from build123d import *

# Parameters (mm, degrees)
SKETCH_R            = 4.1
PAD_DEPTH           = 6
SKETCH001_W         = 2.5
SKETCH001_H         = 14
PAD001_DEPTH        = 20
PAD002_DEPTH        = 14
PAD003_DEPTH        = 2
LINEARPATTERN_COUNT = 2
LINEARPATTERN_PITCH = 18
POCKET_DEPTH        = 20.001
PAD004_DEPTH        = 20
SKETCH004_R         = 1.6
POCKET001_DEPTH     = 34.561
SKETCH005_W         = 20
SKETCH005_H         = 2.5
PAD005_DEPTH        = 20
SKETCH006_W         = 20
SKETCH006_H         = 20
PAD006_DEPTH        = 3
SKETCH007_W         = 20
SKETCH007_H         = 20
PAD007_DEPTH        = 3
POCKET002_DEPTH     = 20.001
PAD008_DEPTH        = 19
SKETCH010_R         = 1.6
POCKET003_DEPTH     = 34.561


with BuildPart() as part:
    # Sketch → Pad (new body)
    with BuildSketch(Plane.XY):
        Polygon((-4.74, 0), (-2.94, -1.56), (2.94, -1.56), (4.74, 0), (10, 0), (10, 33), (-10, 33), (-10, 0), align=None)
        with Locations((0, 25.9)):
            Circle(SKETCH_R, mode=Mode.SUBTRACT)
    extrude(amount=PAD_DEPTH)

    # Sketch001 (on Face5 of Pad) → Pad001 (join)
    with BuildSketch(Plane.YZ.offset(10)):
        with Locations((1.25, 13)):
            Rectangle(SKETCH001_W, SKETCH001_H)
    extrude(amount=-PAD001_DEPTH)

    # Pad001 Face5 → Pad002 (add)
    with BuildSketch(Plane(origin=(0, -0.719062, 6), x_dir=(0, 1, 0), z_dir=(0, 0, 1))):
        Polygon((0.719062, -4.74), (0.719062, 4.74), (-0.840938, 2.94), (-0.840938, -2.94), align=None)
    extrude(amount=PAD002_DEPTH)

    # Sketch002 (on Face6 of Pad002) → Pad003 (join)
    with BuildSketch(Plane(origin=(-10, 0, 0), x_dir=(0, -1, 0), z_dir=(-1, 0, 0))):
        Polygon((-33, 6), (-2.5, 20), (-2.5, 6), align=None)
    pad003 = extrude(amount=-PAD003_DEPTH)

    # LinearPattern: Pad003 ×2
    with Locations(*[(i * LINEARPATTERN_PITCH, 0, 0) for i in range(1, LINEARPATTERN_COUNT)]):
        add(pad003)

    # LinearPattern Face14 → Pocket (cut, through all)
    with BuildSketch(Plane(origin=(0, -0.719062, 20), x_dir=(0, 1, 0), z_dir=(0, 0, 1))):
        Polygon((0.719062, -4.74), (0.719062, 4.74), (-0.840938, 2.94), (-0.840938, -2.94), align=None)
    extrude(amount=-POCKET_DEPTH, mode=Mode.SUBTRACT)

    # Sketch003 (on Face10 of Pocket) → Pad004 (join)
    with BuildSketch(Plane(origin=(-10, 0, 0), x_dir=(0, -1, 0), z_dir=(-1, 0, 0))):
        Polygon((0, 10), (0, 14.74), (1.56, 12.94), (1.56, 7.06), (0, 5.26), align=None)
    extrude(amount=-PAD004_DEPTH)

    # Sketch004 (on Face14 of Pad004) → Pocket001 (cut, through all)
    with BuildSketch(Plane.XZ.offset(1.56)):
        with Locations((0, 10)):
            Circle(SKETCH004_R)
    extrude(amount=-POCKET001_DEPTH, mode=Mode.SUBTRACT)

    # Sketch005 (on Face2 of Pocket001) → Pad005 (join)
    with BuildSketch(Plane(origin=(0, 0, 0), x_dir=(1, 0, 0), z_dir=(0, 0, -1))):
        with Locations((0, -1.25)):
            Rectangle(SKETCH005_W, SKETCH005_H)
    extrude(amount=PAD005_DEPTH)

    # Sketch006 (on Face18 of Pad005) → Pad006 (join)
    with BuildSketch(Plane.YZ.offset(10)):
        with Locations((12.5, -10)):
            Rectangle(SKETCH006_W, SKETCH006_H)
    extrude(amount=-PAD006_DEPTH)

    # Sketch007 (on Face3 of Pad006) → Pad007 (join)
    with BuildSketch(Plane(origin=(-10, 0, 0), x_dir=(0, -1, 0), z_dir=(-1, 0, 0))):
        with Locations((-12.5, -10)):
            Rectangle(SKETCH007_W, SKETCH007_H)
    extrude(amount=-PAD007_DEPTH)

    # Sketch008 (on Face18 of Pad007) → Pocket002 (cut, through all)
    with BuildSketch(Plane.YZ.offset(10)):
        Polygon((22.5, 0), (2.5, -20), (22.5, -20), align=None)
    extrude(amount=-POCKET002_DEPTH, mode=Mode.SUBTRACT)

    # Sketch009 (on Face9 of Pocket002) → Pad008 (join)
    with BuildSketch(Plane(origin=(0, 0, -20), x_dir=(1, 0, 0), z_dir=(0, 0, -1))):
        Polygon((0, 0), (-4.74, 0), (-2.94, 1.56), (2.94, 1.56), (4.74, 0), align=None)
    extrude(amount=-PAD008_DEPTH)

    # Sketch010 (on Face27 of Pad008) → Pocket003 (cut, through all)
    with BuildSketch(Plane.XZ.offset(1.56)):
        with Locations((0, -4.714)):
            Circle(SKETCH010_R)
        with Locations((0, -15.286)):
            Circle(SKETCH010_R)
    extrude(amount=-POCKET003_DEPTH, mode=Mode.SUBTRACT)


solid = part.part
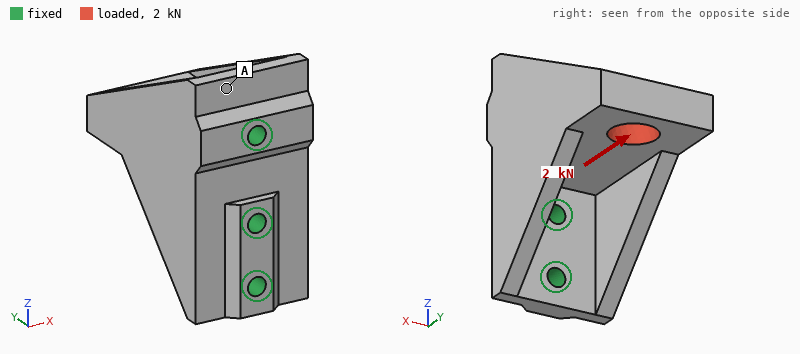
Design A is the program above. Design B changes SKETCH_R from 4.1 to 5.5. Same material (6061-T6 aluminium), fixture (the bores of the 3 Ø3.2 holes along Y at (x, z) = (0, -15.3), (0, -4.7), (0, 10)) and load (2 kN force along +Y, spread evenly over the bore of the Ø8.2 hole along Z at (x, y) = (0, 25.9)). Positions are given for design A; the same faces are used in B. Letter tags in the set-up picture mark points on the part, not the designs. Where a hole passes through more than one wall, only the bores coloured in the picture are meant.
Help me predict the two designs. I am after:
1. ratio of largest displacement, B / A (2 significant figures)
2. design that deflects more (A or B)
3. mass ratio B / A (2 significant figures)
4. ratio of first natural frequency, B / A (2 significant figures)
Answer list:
1.4
B
0.97
1.0
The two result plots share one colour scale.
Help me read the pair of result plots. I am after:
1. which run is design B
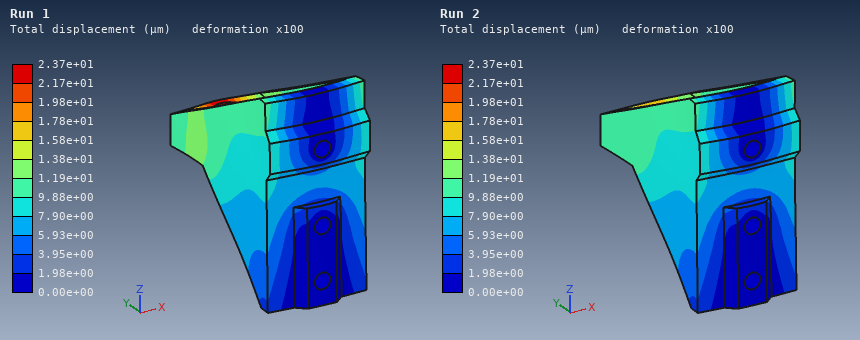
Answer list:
Run 1
